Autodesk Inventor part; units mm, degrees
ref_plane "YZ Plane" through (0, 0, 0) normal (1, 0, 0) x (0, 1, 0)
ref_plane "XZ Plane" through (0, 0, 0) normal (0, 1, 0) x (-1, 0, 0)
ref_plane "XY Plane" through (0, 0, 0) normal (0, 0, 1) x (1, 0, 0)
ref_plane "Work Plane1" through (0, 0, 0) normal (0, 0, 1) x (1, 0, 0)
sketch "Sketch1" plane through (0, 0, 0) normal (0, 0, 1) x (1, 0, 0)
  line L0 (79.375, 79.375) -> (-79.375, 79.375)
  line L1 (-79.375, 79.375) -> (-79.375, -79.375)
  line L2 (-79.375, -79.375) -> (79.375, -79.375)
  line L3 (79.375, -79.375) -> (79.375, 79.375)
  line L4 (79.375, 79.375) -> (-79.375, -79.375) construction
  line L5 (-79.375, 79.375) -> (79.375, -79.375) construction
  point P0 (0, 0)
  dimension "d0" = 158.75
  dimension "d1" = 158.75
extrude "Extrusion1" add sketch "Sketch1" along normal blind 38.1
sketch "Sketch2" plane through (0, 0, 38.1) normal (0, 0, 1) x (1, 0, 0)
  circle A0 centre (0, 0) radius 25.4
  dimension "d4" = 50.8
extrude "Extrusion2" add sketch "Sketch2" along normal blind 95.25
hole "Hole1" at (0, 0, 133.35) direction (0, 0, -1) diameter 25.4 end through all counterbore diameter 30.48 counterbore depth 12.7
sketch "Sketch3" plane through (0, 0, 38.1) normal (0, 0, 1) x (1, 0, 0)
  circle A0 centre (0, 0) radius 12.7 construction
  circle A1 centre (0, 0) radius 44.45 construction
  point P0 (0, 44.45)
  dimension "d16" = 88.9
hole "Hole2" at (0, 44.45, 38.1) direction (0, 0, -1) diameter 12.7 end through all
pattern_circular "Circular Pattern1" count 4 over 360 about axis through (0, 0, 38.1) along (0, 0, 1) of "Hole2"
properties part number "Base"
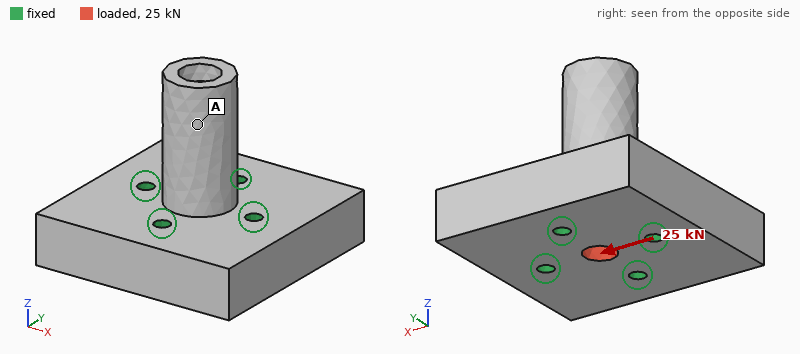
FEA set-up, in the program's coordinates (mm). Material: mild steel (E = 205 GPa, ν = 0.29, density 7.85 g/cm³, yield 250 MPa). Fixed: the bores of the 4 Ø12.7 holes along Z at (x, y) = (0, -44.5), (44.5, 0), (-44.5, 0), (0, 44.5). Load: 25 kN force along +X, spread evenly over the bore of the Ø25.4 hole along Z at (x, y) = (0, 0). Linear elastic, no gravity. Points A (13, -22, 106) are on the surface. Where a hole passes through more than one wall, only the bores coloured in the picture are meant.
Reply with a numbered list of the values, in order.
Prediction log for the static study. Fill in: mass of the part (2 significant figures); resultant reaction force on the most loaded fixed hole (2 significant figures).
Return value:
1. 8.3 kg
2. 14 kN
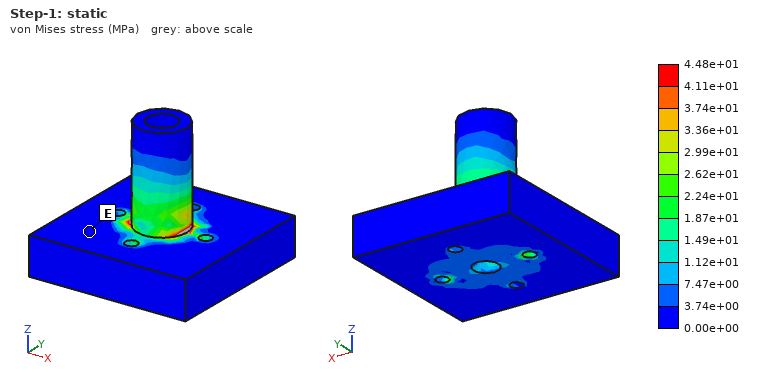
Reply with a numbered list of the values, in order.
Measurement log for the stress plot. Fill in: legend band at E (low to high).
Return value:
1. 0.00e+00 to 3.74e+00 MPa
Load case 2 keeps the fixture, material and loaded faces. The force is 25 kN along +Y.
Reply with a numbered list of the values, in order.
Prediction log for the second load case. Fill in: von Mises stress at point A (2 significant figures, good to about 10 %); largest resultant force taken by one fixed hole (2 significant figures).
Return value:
1. 4.1 MPa
2. 14 kN
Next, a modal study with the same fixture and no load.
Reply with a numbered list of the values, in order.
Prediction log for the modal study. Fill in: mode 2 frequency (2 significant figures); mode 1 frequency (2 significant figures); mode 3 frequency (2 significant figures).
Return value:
1. 3100 Hz
2. 3100 Hz
3. 6200 Hz
